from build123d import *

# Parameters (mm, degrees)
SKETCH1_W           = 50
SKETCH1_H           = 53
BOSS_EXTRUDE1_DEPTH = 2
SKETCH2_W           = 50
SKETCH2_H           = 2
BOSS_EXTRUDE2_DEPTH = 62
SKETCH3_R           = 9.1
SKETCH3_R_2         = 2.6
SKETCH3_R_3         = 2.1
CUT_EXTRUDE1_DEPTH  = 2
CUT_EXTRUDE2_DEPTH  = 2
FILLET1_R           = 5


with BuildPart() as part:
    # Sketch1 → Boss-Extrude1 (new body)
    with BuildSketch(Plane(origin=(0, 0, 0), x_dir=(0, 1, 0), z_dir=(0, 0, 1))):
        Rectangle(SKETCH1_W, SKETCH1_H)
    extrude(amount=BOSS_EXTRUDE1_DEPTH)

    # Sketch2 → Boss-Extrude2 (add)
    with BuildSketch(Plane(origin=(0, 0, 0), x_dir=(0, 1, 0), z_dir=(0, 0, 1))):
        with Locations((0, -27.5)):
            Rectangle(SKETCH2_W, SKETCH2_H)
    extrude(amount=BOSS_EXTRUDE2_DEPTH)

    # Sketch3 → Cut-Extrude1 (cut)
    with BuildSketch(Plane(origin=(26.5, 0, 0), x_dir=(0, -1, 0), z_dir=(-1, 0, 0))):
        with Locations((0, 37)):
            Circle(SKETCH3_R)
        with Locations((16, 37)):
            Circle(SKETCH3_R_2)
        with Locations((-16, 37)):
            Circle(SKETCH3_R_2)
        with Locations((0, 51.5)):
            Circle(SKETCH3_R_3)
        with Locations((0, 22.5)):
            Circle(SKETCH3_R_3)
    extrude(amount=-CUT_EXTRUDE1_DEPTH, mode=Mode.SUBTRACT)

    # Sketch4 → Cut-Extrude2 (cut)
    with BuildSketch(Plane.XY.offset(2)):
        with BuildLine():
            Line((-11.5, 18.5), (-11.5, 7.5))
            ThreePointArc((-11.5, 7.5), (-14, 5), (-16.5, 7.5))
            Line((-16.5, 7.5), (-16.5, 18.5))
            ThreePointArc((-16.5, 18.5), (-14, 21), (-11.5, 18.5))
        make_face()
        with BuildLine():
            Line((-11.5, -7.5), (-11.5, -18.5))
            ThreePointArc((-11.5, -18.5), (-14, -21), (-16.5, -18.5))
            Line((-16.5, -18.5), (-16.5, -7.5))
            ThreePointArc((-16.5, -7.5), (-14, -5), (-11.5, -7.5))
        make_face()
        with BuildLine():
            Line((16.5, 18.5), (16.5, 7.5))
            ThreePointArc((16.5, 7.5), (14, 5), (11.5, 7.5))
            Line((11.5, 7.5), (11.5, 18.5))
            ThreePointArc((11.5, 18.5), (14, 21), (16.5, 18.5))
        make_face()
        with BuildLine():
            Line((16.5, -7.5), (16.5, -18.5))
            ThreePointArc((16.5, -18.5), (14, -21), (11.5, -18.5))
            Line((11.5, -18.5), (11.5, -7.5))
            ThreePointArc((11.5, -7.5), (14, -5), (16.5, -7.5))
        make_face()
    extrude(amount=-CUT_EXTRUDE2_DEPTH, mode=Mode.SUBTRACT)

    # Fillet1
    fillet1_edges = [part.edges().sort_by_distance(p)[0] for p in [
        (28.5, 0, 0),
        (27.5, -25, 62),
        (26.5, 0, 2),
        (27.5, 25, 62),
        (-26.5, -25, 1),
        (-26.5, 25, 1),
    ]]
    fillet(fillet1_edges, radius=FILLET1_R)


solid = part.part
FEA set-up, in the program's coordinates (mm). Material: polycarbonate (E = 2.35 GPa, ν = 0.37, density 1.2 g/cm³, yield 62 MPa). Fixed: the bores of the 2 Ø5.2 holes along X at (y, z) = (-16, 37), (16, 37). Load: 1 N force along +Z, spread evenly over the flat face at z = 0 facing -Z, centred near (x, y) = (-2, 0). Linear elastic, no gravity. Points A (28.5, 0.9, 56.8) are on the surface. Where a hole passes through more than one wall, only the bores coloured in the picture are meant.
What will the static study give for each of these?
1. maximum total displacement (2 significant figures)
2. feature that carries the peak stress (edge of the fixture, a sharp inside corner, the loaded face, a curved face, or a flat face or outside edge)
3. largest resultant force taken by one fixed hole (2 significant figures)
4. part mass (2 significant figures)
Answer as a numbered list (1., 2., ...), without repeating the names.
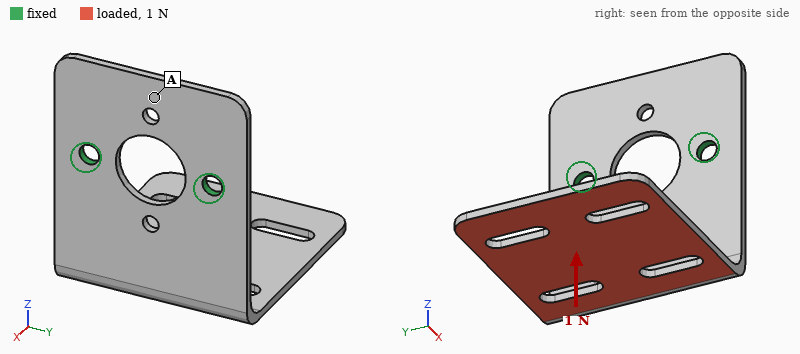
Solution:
1. 1.0 mm
2. a flat face or outside edge
3. 0.54 N
4. 12 g
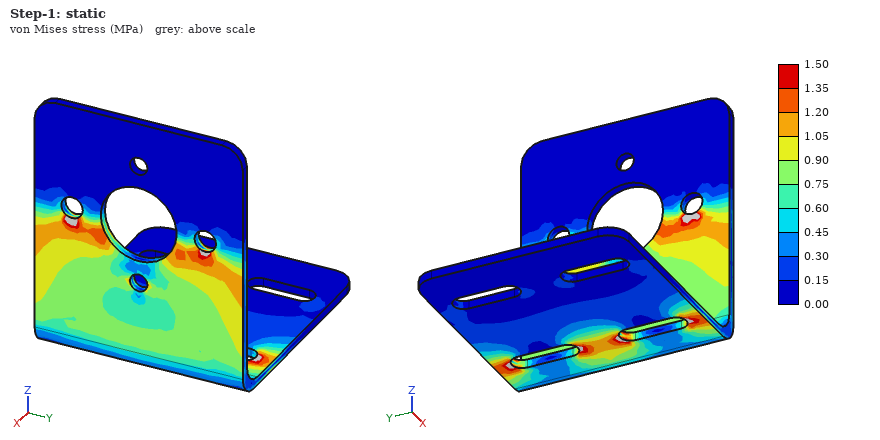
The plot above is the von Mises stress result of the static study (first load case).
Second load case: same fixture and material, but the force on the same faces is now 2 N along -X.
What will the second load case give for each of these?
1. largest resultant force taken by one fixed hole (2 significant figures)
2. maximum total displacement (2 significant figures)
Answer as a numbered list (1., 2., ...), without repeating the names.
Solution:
1. 1.0 N
2. 1.1 mm
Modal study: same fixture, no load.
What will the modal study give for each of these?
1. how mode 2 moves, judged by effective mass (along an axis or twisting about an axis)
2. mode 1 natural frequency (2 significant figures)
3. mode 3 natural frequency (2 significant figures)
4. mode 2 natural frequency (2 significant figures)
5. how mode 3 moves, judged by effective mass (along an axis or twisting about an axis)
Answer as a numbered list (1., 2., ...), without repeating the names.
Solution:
1. along Y
2. 76 Hz
3. 220 Hz
4. 160 Hz
5. along X
